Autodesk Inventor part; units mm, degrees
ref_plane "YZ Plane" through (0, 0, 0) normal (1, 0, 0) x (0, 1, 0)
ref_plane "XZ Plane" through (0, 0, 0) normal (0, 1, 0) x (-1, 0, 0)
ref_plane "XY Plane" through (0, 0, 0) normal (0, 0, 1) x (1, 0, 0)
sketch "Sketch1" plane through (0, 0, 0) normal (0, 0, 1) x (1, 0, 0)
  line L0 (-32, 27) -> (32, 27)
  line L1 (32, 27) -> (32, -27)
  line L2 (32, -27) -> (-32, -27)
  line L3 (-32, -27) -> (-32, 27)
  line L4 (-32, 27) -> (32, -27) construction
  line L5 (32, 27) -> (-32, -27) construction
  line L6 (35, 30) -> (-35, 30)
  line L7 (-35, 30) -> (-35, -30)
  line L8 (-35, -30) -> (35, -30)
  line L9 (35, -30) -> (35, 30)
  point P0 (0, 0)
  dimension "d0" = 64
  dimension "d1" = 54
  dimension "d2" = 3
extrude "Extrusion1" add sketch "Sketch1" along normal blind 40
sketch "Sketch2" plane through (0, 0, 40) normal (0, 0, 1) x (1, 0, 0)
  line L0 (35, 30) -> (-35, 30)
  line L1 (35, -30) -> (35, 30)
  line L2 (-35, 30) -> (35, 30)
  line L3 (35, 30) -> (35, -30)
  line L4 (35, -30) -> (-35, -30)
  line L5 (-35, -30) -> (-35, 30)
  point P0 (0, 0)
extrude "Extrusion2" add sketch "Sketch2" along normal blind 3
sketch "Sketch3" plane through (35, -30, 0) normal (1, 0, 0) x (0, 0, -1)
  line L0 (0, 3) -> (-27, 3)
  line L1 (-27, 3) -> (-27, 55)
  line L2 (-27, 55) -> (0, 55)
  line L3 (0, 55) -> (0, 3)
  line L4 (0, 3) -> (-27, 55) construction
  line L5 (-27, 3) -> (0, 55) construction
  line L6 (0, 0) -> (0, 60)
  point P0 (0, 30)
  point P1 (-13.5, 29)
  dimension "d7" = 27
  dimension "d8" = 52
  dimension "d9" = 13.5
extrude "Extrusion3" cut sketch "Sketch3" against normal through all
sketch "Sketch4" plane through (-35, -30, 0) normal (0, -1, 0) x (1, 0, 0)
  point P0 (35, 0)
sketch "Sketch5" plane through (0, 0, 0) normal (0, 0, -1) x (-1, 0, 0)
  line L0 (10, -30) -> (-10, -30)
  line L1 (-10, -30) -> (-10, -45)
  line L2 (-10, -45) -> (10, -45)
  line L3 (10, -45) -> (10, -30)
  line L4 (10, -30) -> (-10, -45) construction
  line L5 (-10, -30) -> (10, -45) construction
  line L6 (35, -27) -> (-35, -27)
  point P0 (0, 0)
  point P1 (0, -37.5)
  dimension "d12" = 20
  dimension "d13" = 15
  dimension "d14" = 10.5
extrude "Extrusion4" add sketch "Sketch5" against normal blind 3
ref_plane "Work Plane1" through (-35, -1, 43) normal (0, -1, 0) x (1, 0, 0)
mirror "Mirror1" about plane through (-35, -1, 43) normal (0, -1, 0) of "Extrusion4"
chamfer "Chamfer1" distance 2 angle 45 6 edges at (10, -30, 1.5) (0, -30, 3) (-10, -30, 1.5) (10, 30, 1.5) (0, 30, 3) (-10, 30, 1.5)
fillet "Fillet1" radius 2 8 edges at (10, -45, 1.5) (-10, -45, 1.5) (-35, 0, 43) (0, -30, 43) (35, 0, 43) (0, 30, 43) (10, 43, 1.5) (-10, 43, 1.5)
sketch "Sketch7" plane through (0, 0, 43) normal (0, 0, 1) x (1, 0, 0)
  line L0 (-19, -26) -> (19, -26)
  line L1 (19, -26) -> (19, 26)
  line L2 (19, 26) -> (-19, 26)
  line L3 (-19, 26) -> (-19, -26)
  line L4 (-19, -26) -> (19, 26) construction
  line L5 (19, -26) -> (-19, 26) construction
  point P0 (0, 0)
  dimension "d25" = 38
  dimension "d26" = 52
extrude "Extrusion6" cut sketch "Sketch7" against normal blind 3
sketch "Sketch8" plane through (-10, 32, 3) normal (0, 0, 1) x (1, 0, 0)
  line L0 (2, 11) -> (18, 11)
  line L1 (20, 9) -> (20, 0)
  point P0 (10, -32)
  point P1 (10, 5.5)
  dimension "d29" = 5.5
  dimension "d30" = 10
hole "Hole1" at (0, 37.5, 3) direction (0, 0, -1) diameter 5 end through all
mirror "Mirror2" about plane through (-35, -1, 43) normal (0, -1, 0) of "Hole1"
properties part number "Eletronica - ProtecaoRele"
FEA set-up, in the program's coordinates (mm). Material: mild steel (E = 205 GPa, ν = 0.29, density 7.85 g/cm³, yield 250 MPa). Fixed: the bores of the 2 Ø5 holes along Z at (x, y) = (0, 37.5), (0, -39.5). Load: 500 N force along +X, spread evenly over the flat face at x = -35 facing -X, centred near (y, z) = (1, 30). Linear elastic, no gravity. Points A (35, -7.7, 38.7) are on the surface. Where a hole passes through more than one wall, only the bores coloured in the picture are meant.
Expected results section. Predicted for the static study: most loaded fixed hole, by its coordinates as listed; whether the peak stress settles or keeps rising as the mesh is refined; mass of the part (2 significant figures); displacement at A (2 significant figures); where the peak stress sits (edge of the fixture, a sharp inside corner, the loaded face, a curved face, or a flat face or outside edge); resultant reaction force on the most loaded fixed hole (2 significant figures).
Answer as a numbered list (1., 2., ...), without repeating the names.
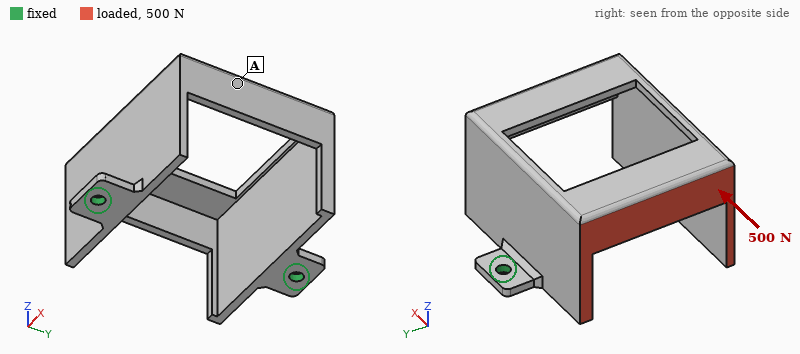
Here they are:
1. (0, 37.5)
2. keeps rising
3. 230 g
4. 0.14 mm
5. edge of the fixture
6. 270 N
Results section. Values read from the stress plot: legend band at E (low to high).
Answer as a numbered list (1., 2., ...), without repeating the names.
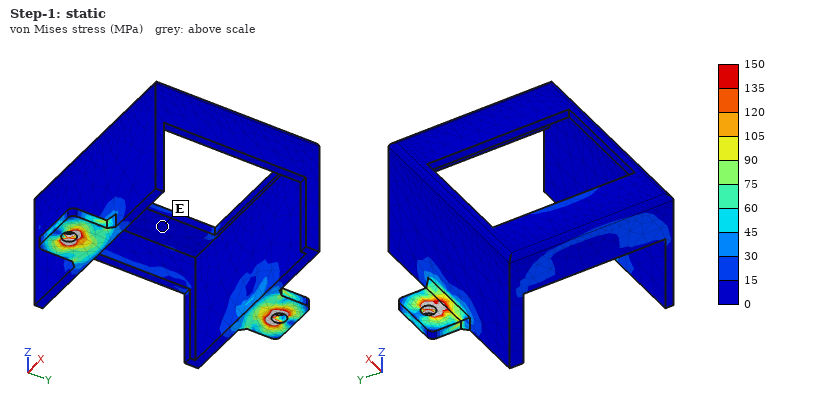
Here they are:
1. 0 to 15 MPa
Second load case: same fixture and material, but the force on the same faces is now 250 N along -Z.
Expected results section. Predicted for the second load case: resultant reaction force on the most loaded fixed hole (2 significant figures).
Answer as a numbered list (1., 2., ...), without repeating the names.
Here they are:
1. 130 N
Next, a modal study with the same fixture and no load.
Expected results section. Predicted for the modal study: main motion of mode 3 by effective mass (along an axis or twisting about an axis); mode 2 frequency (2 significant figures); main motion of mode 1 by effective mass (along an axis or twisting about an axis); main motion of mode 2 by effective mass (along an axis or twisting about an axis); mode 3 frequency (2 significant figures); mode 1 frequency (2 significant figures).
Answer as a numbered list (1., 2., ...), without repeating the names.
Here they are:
1. twisting about Z
2. 1100 Hz
3. along X
4. along Y
5. 1300 Hz
6. 660 Hz
